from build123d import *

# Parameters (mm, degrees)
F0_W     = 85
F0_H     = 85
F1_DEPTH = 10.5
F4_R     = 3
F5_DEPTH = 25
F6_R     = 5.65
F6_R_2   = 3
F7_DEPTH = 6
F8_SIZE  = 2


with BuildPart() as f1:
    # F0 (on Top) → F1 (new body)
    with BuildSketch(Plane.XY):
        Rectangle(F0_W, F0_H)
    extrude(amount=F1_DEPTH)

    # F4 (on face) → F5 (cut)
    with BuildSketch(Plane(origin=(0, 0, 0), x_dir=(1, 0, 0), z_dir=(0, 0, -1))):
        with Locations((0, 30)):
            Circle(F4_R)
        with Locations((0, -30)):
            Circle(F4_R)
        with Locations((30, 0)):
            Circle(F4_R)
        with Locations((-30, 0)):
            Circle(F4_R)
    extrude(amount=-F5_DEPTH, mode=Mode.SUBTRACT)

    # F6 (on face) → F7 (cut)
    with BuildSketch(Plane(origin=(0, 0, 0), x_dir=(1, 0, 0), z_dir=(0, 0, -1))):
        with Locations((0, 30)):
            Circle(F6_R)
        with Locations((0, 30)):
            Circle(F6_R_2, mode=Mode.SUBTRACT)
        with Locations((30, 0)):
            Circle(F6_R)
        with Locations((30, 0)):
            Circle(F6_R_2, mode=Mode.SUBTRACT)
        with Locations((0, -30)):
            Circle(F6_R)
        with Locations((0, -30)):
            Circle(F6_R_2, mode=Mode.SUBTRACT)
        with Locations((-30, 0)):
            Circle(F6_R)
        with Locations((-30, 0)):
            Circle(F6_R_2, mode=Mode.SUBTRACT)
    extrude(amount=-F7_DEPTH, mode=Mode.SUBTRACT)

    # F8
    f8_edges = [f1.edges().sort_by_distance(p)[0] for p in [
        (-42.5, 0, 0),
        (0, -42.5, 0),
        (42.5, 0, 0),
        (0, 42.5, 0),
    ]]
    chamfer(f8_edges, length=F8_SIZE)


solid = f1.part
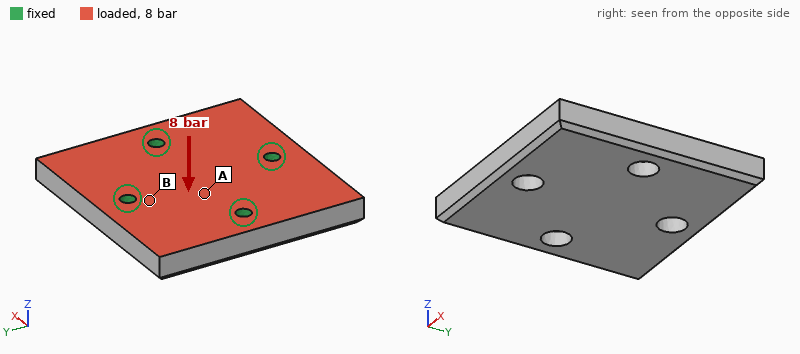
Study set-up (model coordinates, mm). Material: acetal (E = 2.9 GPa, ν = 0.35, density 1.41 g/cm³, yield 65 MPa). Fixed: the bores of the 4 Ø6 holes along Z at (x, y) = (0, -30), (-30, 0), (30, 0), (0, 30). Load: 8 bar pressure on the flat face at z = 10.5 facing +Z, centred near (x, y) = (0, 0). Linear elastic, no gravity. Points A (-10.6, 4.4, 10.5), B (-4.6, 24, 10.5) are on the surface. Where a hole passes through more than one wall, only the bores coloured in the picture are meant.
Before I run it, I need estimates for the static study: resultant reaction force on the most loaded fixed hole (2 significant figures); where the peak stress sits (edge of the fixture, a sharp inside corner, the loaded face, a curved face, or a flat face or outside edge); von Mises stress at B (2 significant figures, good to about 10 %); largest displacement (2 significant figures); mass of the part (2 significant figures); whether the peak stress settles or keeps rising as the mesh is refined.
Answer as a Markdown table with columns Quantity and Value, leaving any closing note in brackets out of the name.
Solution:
| Quantity | Value |
|---|---|
| resultant reaction force on the most loaded fixed hole | 1.4 kN |
| where the peak stress sits | edge of the fixture |
| von Mises stress at B | 11 MPa |
| largest displacement | 0.57 mm |
| mass of the part | 100 g |
| whether the peak stress settles or keeps rising as the mesh is refined | keeps rising |
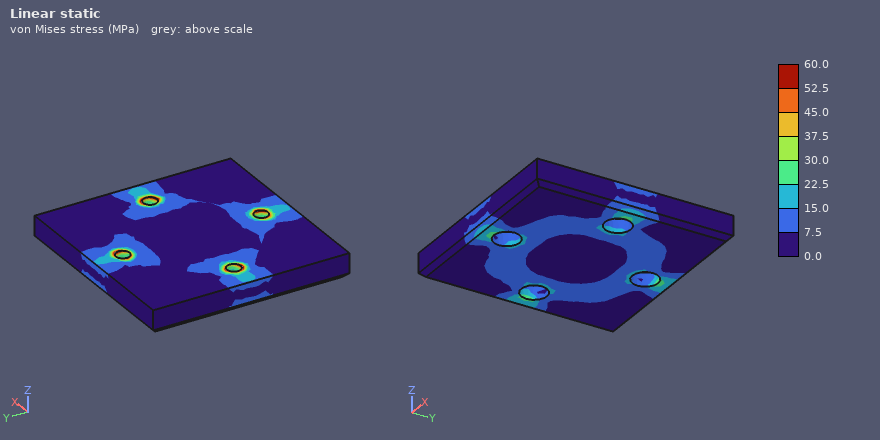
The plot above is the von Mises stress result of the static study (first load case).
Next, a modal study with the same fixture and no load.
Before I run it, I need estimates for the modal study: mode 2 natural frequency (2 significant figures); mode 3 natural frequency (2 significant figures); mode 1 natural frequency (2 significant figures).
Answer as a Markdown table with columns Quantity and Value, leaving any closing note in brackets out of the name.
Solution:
| Quantity | Value |
|---|---|
| mode 2 natural frequency | 1900 Hz |
| mode 3 natural frequency | 1900 Hz |
| mode 1 natural frequency | 1700 Hz |
